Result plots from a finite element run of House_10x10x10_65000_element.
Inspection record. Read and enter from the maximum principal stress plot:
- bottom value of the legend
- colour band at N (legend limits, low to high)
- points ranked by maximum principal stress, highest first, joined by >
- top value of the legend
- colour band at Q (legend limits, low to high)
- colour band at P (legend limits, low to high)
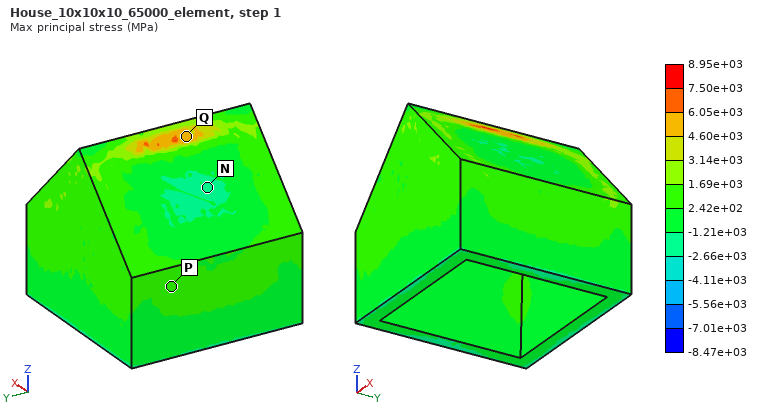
-8.47e+03 MPa
-2.66e+03 to -1.21e+03 MPa
Q > P > N
8.95e+03 MPa
4.60e+03 to 6.05e+03 MPa
2.42e+02 to 1.69e+03 MPa
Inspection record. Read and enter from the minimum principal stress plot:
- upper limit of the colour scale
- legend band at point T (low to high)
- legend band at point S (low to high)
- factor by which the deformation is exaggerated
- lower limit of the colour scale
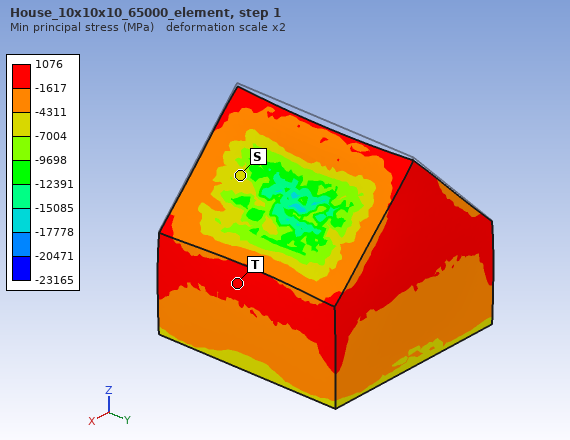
1076 MPa
-1617 to 1076 MPa
-7004 to -4311 MPa
2
-23165 MPa
